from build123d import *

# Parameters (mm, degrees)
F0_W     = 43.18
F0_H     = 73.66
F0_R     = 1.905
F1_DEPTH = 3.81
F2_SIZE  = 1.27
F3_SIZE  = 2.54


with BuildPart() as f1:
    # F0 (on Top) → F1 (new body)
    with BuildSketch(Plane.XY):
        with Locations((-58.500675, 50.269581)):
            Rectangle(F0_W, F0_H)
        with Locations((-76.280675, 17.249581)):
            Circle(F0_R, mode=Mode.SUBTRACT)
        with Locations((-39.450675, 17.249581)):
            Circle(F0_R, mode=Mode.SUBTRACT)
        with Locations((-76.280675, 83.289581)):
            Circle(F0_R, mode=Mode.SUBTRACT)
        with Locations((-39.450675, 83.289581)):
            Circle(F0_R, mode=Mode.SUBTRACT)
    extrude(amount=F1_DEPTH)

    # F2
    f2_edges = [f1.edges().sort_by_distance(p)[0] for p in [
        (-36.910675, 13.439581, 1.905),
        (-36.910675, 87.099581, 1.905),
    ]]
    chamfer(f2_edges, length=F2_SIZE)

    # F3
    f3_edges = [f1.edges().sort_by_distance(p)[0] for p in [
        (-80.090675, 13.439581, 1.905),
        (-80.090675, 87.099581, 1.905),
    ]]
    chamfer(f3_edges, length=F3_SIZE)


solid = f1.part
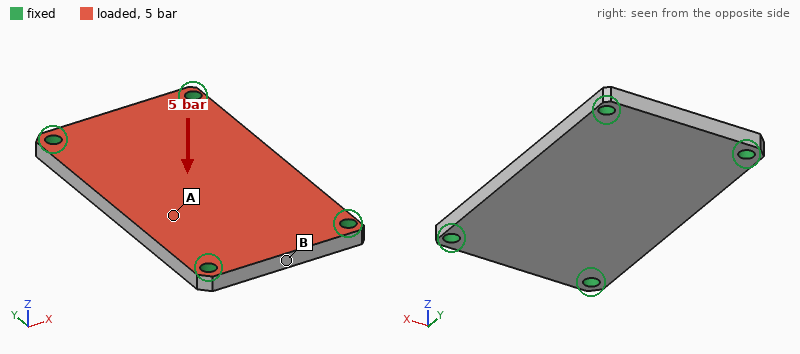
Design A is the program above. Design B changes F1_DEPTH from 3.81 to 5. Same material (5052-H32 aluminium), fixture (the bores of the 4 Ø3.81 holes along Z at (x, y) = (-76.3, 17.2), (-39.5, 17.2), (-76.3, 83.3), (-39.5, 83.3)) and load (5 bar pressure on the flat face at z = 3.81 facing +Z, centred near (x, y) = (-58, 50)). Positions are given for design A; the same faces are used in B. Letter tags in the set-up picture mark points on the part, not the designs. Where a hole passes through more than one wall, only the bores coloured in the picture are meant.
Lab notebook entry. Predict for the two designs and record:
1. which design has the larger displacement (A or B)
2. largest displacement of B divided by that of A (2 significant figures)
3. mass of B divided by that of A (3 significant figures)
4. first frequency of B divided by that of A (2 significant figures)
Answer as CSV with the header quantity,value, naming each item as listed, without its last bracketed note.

quantity,value
which design has the larger displacement,A
largest displacement of B divided by that of A,0.47
mass of B divided by that of A,1.31
first frequency of B divided by that of A,1.3
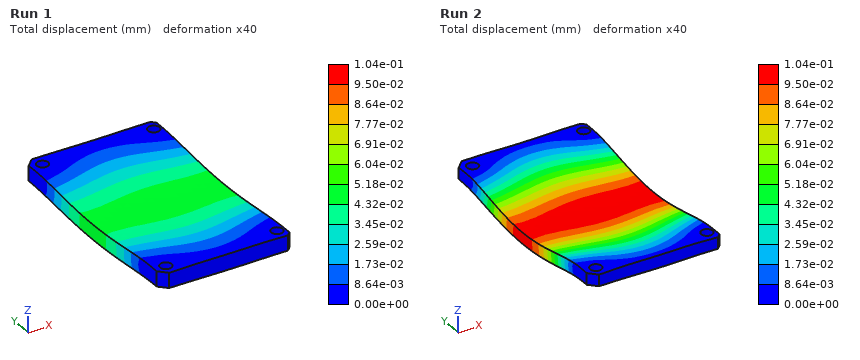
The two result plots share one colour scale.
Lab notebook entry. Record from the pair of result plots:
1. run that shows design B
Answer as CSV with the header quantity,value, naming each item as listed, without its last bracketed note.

quantity,value
run that shows design B,Run 1
